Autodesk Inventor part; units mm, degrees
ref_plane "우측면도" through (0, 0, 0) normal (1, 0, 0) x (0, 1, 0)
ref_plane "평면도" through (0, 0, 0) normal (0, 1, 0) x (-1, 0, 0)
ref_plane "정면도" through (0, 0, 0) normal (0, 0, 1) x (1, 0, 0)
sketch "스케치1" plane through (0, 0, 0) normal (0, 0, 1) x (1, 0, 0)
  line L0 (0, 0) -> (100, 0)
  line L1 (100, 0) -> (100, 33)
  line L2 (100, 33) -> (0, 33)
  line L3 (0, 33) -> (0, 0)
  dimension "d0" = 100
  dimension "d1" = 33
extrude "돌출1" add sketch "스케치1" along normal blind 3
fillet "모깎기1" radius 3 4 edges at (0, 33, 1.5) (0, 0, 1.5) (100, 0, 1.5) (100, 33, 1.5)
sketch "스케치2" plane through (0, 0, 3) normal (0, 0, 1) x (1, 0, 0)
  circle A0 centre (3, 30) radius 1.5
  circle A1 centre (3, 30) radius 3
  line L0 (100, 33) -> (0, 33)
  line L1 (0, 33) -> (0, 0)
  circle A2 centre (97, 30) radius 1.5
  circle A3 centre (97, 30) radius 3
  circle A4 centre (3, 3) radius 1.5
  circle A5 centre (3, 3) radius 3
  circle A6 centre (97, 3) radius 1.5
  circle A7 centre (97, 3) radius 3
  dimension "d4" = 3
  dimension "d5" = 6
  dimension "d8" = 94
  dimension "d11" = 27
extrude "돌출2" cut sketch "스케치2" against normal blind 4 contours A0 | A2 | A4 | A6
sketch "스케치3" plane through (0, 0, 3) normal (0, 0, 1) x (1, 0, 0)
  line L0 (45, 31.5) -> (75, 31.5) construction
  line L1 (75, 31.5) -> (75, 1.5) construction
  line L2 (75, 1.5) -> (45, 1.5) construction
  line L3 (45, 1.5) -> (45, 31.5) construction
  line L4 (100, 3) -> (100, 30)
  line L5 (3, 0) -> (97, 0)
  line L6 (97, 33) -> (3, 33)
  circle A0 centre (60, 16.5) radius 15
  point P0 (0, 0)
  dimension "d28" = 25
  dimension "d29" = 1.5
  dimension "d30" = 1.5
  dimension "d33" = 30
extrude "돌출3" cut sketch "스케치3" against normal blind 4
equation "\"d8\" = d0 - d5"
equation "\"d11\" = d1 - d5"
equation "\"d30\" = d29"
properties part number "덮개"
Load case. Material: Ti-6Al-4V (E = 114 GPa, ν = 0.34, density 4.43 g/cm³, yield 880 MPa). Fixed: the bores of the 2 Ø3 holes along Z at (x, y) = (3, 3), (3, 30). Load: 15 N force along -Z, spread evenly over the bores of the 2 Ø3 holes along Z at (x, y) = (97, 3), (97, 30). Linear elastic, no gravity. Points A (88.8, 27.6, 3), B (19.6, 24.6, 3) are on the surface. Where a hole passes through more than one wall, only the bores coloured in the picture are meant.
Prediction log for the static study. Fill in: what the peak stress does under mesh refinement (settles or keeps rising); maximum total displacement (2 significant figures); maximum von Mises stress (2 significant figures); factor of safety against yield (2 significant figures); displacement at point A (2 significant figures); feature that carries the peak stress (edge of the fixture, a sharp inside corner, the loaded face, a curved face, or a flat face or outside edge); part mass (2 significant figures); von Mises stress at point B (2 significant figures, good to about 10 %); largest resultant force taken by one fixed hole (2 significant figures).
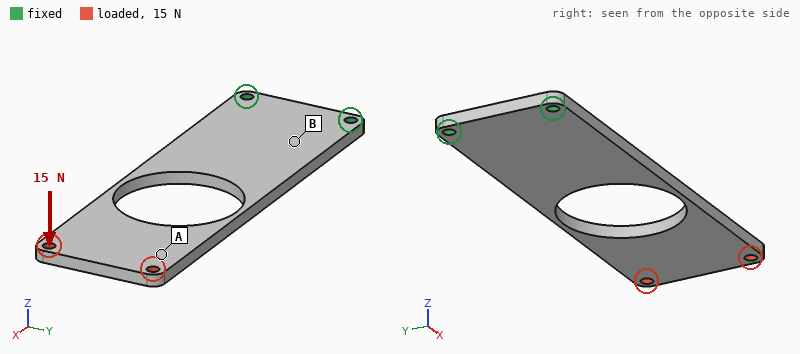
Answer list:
settles
0.97 mm
130 MPa
6.6
0.76 mm
a curved face
34 g
23 MPa
7.5 N
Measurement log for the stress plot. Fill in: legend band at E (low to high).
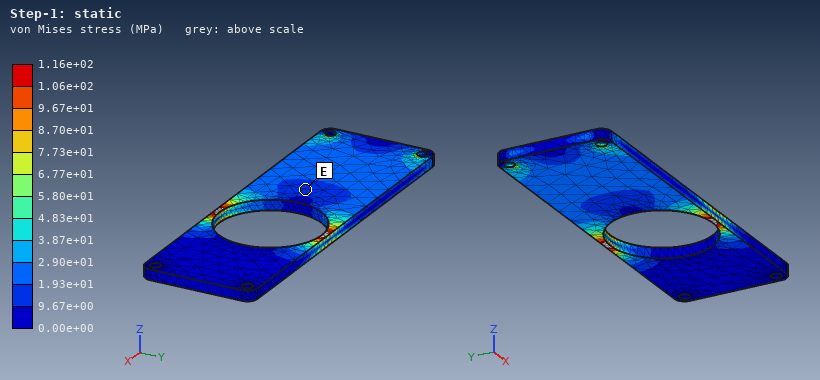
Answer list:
9.67e+00 to 1.93e+01 MPa
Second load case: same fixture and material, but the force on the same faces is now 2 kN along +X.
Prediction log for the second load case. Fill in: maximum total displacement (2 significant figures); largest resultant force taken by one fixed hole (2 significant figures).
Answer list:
73 µm
1.0 kN
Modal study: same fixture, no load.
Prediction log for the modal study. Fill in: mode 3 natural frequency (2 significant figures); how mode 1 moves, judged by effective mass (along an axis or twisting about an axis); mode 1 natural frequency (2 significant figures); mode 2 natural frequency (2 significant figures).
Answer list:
1300 Hz
along Z
230 Hz
1300 Hz
